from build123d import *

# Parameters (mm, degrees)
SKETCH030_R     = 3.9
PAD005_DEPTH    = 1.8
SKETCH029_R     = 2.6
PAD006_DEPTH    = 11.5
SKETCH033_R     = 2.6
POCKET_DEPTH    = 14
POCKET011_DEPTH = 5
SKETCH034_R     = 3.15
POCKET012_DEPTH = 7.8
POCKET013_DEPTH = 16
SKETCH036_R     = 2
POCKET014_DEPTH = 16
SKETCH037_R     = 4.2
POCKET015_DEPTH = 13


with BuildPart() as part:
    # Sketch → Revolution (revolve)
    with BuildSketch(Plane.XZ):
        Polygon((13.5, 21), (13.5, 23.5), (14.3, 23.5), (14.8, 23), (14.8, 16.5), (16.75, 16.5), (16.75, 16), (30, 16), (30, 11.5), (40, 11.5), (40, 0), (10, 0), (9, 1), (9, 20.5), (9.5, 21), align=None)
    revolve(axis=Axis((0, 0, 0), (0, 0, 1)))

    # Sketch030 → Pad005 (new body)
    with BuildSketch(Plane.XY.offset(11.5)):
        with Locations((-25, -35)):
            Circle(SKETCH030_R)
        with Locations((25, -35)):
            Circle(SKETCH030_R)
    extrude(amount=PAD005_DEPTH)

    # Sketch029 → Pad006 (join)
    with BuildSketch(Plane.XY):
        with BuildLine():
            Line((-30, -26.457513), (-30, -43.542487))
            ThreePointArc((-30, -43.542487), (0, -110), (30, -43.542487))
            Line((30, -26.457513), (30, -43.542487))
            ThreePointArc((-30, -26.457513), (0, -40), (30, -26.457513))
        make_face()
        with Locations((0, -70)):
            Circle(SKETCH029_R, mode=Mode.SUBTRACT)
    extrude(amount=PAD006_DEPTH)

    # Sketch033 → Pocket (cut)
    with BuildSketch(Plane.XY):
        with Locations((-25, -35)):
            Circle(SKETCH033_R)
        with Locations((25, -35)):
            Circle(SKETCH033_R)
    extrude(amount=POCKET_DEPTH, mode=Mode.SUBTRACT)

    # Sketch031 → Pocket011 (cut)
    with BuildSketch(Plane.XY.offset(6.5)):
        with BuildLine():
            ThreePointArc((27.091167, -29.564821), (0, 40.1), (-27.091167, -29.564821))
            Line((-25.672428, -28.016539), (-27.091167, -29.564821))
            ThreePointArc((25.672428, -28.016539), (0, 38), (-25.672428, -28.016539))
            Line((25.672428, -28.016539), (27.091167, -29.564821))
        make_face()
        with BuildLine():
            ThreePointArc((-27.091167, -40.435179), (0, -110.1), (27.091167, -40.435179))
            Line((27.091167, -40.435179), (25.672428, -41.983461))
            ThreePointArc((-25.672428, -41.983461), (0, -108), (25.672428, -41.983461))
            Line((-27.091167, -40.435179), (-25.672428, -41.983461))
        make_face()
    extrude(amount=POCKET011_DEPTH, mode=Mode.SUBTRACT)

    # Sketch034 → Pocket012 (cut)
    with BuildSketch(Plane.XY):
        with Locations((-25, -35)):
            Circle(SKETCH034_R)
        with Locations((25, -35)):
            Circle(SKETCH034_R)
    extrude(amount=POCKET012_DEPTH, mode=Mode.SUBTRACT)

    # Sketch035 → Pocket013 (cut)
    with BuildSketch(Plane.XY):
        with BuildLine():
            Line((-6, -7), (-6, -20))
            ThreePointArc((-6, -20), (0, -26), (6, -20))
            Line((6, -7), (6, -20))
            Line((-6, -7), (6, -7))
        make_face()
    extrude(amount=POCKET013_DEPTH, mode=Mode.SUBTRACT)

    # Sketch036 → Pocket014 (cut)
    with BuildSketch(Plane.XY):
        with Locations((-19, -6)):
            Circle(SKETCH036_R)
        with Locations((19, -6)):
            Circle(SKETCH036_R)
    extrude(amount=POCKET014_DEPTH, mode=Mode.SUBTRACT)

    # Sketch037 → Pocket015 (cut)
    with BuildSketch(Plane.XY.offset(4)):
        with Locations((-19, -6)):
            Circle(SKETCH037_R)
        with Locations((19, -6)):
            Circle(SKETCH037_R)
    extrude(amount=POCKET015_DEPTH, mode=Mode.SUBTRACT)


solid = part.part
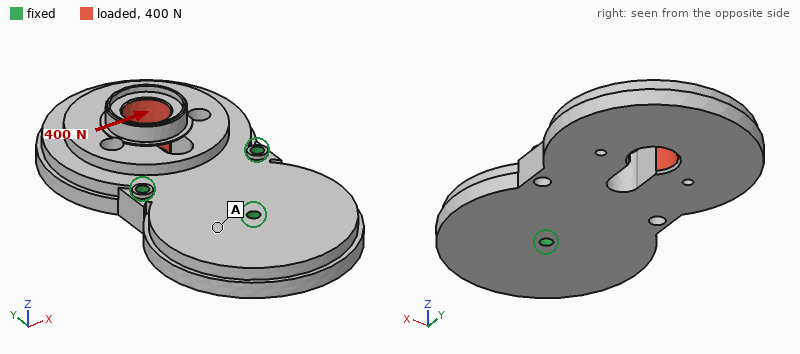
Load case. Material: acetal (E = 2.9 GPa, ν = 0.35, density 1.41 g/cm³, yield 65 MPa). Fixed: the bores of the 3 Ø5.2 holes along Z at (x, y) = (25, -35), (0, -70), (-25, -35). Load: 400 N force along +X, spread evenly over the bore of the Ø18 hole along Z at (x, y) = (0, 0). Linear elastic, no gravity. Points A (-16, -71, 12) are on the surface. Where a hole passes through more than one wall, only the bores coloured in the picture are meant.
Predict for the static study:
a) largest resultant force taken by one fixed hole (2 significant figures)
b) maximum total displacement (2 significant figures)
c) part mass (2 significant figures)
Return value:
340 N
0.12 mm
160 g
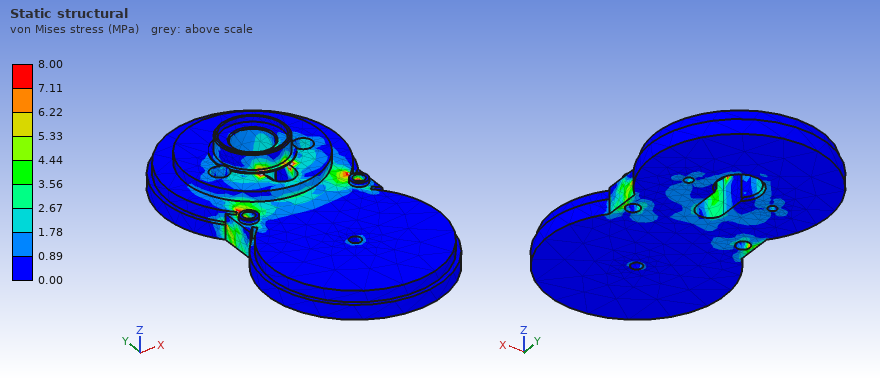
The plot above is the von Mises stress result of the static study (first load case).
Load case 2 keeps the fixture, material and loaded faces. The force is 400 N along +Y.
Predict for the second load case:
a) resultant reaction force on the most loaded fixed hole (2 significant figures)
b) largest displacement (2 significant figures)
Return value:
160 N
0.16 mm
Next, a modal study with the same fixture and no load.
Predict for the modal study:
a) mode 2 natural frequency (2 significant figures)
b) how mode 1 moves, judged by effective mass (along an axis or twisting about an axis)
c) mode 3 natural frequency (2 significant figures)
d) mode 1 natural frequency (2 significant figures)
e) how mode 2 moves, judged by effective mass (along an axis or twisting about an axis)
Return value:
1200 Hz
along Z
1200 Hz
390 Hz
along X
